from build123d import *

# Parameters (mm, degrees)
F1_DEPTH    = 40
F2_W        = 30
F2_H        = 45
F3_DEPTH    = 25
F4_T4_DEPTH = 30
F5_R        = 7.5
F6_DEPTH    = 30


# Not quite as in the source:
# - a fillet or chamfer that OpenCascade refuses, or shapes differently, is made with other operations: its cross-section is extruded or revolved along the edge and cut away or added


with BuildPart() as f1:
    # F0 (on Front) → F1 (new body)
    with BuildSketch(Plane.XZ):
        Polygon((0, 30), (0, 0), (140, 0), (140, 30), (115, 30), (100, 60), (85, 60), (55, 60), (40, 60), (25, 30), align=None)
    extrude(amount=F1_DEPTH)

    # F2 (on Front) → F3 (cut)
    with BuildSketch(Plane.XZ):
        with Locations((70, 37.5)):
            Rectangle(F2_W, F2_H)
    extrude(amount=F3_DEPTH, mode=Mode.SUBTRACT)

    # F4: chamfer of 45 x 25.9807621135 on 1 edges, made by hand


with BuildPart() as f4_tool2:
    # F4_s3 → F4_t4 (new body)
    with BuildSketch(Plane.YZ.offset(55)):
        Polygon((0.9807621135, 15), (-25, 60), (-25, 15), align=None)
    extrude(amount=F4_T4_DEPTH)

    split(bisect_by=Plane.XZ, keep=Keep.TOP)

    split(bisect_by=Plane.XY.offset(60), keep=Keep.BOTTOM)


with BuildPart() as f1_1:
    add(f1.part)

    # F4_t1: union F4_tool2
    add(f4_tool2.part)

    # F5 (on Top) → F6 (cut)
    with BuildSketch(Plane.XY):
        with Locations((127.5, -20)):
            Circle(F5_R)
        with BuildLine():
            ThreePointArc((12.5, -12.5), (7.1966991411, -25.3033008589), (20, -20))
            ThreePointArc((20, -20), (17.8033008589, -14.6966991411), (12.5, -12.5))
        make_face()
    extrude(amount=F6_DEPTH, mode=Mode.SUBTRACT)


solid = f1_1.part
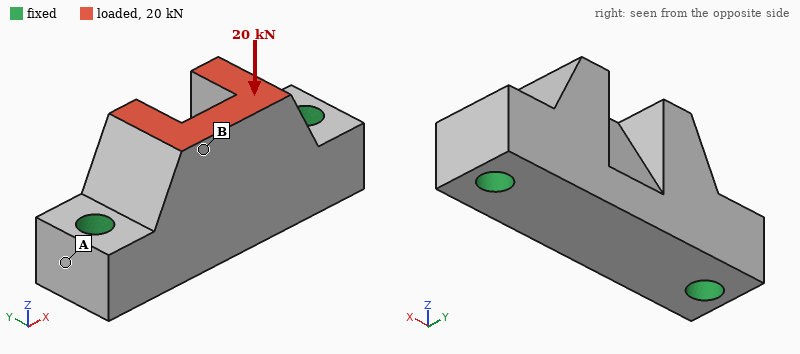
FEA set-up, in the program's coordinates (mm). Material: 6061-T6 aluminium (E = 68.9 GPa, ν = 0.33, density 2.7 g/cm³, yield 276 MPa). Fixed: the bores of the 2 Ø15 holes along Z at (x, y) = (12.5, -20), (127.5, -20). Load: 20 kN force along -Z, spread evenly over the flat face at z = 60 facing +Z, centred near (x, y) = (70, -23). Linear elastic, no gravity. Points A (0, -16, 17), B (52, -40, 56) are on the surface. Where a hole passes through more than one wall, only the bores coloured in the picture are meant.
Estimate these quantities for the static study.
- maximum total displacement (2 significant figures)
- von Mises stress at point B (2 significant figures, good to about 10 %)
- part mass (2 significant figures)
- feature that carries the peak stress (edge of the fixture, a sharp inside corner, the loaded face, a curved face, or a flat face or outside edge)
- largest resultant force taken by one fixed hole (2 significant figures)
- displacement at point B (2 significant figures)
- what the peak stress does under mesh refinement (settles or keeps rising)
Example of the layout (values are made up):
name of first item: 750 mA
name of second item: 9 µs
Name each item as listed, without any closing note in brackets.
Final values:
maximum total displacement: 28 µm
von Mises stress at point B: 12 MPa
part mass: 620 g
feature that carries the peak stress: edge of the fixture
largest resultant force taken by one fixed hole: 11 kN
displacement at point B: 24 µm
what the peak stress does under mesh refinement: keeps rising
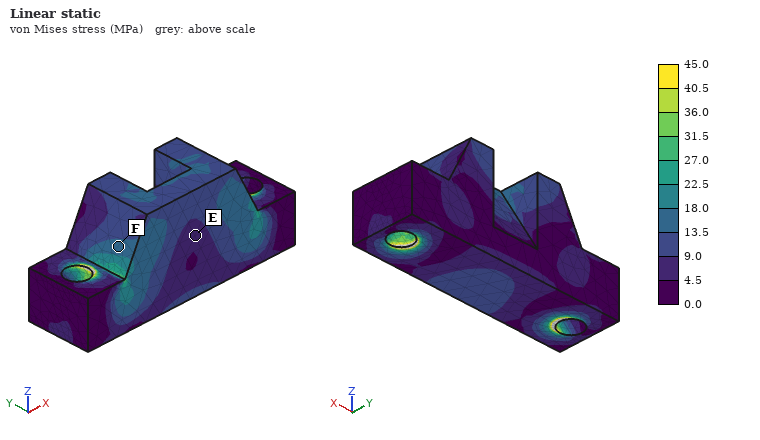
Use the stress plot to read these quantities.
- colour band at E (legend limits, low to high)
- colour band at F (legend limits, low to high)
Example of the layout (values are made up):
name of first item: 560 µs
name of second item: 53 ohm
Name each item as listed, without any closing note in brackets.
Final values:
colour band at E: 4.5 to 9.0 MPa
colour band at F: 13.5 to 18.0 MPa
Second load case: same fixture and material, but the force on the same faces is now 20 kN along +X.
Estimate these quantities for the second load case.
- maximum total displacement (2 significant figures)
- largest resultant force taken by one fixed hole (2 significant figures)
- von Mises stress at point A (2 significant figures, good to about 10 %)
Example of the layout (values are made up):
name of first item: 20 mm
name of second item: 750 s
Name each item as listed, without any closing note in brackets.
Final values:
maximum total displacement: 34 µm
largest resultant force taken by one fixed hole: 13 kN
von Mises stress at point A: 4.1 MPa
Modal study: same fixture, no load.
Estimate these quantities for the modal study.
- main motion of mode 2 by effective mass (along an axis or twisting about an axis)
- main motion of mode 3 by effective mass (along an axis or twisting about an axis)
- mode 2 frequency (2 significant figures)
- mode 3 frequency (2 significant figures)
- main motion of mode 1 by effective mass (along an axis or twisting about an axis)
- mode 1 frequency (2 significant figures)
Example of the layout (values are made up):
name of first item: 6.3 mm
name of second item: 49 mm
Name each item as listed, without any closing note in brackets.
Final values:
main motion of mode 2 by effective mass: along Z
main motion of mode 3 by effective mass: along Y
mode 2 frequency: 8900 Hz
mode 3 frequency: 9700 Hz
main motion of mode 1 by effective mass: along Y
mode 1 frequency: 5800 Hz
